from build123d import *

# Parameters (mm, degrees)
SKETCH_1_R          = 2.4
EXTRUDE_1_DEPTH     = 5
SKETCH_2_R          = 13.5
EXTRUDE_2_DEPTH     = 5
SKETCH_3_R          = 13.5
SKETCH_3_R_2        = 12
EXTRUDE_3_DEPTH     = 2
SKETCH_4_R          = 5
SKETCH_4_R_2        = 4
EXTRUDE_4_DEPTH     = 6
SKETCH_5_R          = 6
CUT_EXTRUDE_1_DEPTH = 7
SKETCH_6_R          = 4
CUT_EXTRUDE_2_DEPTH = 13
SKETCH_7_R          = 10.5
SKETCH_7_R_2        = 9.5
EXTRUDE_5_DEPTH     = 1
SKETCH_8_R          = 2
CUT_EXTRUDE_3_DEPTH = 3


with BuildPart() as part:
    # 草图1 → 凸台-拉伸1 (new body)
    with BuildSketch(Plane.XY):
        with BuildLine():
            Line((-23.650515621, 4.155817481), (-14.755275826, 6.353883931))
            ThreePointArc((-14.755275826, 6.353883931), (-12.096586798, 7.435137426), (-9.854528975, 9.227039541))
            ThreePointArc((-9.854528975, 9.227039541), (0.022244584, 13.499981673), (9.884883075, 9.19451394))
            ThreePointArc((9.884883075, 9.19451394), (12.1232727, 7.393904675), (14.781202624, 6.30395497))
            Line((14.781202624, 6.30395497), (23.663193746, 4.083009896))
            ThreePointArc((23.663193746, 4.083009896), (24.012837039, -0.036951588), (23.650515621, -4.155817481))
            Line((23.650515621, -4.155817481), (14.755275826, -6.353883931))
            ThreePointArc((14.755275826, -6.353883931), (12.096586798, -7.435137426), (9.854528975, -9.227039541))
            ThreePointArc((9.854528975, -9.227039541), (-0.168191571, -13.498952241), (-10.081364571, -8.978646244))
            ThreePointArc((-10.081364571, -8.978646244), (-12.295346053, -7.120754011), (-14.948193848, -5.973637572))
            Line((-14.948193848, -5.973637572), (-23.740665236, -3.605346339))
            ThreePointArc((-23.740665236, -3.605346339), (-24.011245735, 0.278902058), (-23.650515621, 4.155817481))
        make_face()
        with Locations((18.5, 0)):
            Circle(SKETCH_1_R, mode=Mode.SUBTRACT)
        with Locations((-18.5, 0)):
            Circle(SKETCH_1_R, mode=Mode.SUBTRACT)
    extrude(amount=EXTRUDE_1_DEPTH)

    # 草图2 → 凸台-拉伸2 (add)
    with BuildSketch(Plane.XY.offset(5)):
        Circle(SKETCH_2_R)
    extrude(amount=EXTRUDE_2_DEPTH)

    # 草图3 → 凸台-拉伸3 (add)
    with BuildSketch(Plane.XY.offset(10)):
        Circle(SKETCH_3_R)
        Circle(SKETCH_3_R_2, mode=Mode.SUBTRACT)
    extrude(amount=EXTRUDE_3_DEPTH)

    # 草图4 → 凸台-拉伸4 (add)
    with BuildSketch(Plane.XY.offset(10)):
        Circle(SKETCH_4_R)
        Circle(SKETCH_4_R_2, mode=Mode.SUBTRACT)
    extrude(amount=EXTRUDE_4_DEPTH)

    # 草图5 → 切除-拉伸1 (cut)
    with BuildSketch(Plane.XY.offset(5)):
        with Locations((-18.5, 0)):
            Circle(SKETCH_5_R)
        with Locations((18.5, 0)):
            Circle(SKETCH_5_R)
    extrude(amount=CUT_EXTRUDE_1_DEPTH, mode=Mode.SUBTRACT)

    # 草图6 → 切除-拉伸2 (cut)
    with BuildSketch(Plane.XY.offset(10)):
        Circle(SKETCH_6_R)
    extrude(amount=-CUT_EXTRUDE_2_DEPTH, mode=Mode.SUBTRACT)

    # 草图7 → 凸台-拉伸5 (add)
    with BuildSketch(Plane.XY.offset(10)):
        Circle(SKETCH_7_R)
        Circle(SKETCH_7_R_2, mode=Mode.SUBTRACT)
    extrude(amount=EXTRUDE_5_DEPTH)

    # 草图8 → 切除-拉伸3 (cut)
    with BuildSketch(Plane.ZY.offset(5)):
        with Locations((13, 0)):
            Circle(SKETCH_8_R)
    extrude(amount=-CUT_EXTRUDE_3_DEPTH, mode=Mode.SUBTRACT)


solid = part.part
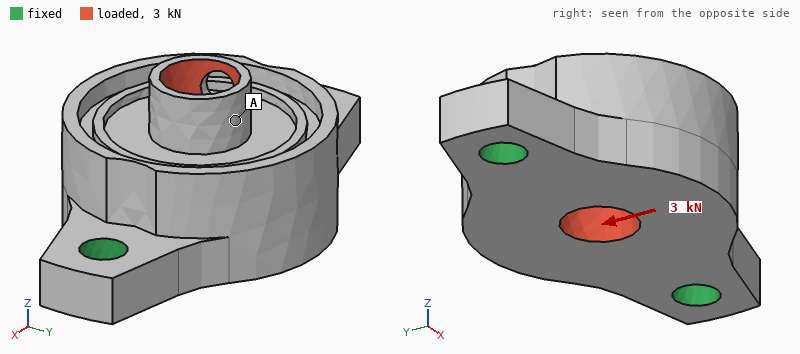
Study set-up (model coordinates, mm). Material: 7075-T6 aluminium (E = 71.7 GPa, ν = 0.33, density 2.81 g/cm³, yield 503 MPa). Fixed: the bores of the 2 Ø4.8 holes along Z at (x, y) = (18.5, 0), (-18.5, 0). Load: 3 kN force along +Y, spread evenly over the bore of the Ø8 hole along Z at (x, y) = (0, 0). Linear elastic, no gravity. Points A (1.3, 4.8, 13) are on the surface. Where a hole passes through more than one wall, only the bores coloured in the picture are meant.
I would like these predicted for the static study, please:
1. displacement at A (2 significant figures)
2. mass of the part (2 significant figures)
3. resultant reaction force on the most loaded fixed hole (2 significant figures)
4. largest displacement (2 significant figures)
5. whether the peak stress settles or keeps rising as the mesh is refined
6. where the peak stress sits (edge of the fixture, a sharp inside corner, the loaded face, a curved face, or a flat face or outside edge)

66 µm
19 g
1.5 kN
90 µm
keeps rising
edge of the fixture
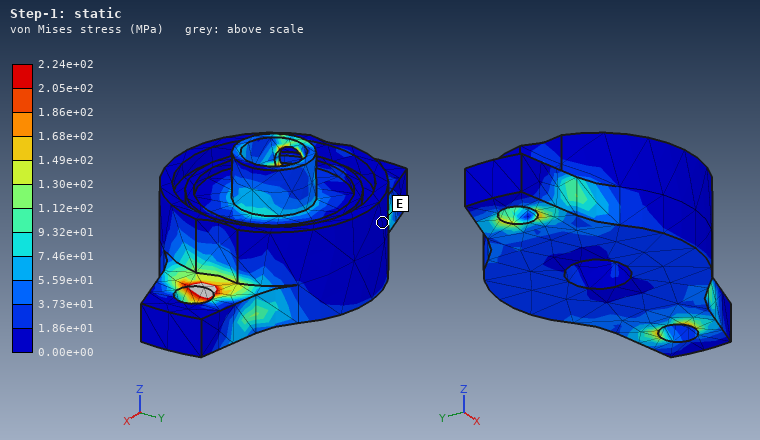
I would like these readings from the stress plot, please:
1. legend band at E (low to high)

0.00e+00 to 1.86e+01 MPa
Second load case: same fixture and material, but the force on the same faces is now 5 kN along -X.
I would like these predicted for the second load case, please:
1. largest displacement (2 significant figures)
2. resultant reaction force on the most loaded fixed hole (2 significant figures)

38 µm
2.7 kN
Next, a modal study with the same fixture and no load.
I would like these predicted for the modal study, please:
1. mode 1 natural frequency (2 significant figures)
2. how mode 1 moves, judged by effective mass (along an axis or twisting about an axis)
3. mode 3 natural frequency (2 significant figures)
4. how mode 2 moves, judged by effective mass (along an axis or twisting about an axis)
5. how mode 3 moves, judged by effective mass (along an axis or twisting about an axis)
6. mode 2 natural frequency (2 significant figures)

9600 Hz
along Y
25 kHz
along Z
along Y
16 kHz
